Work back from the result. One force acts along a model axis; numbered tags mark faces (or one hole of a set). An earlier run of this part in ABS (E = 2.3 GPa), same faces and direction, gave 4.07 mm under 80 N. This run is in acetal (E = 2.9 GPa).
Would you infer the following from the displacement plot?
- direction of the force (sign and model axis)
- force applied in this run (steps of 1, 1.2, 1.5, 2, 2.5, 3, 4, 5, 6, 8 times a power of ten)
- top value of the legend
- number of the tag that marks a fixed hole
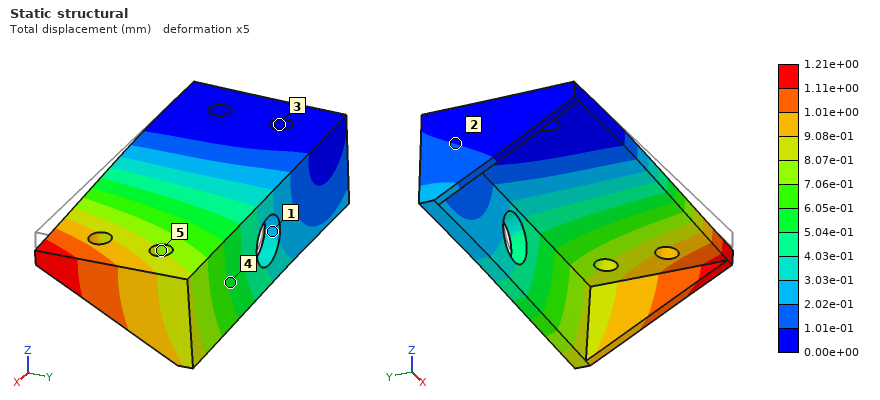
-Z
30 N
1.21e+00 mm
3
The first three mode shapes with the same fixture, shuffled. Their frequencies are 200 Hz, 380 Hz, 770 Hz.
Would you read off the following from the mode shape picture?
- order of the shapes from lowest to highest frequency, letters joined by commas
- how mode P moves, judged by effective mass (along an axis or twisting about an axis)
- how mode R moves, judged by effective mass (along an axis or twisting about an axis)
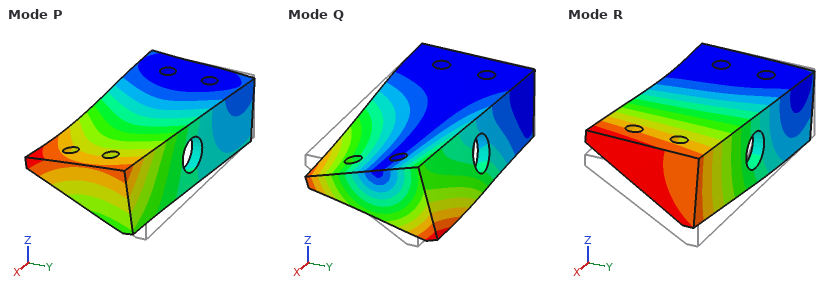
R, Q, P
along Y
along Z
